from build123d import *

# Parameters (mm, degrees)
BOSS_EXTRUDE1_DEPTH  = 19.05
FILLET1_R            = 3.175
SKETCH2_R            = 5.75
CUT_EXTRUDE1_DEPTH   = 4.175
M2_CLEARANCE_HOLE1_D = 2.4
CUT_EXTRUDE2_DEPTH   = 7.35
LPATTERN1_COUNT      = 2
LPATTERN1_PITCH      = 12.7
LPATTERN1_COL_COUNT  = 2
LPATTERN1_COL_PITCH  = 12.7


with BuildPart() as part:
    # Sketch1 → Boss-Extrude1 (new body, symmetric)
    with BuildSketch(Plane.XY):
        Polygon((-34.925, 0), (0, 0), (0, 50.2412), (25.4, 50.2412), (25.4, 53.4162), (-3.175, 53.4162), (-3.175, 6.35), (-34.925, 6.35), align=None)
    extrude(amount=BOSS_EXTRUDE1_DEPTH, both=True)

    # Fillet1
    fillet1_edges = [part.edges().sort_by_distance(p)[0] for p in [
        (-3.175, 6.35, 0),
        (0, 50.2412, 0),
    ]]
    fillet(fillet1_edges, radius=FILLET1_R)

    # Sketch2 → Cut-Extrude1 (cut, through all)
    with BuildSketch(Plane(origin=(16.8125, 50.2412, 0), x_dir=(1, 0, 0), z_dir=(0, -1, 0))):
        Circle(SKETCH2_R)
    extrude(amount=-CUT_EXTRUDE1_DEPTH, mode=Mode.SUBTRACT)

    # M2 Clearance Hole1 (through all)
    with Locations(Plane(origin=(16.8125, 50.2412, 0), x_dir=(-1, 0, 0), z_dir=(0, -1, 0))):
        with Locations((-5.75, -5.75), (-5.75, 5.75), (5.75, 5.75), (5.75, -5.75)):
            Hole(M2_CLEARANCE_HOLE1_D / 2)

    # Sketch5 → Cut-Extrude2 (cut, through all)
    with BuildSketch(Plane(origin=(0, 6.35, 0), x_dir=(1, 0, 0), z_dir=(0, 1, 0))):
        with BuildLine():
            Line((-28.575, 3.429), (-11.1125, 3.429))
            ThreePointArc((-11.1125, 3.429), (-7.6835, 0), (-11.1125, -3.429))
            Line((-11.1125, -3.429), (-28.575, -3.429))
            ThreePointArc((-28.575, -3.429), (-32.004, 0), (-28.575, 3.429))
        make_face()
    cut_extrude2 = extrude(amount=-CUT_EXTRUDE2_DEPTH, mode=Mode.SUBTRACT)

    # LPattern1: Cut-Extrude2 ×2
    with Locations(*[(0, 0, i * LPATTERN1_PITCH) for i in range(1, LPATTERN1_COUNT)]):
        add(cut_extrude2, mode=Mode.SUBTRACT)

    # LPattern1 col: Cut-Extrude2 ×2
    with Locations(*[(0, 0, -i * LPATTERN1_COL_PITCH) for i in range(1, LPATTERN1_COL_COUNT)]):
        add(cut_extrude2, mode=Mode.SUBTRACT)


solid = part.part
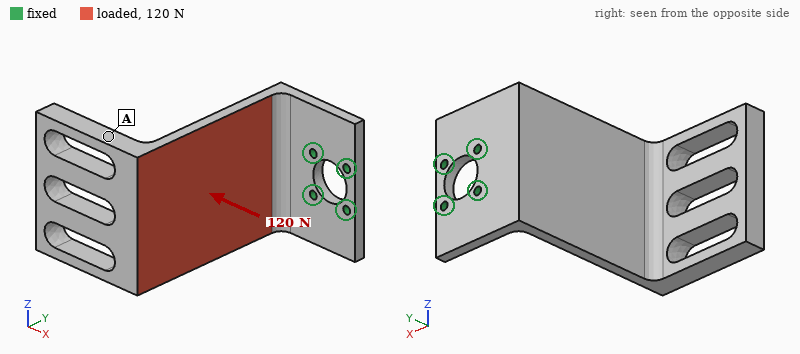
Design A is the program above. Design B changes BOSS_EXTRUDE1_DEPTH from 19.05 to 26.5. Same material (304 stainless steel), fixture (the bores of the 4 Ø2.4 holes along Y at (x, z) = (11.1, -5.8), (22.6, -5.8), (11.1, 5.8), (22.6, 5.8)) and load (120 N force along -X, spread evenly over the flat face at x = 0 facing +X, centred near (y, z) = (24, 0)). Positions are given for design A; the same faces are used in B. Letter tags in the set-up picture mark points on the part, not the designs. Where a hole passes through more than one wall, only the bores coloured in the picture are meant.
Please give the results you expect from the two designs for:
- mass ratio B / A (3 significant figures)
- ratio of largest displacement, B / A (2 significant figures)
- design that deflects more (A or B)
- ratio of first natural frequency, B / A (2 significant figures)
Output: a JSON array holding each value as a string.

["1.49", "0.76", "A", "0.92"]
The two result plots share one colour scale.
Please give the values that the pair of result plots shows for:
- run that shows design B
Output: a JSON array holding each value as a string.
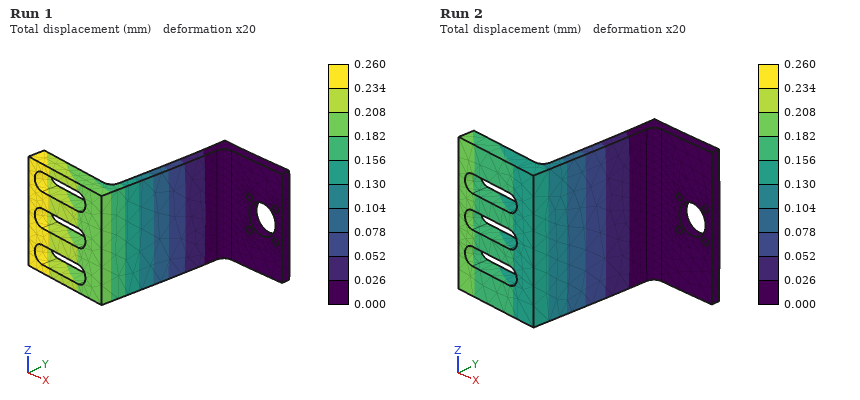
["Run 2"]
